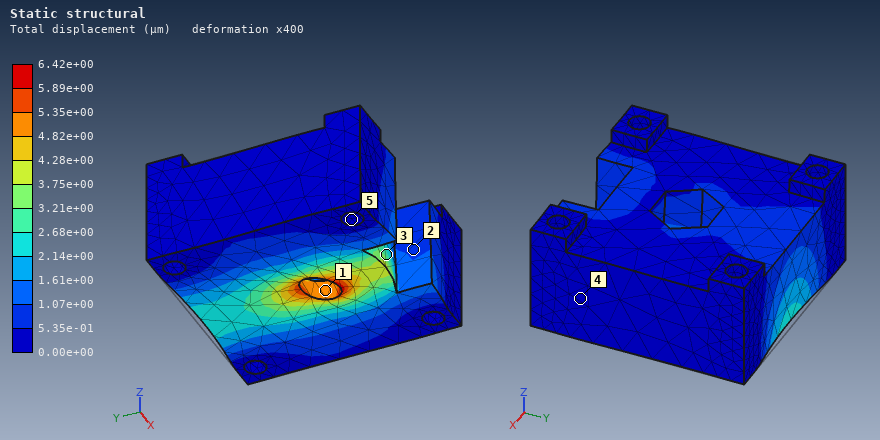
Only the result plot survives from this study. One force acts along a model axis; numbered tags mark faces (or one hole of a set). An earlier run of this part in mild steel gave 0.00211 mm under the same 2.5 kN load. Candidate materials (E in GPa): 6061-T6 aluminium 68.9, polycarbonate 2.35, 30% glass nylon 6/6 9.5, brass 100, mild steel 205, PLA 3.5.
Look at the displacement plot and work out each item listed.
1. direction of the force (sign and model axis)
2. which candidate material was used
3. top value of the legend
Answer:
-Y
6061-T6 aluminium
6.42e+00 µm
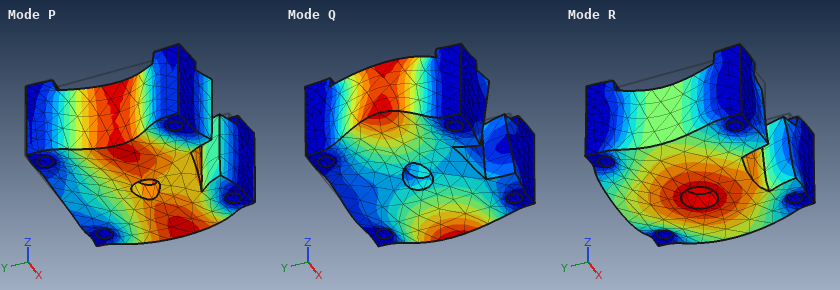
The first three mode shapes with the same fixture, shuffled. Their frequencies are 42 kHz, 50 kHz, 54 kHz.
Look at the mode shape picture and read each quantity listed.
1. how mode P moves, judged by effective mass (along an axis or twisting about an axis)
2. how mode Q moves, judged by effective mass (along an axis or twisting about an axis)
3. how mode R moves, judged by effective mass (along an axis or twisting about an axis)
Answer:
along X
twisting about Y
along Z
